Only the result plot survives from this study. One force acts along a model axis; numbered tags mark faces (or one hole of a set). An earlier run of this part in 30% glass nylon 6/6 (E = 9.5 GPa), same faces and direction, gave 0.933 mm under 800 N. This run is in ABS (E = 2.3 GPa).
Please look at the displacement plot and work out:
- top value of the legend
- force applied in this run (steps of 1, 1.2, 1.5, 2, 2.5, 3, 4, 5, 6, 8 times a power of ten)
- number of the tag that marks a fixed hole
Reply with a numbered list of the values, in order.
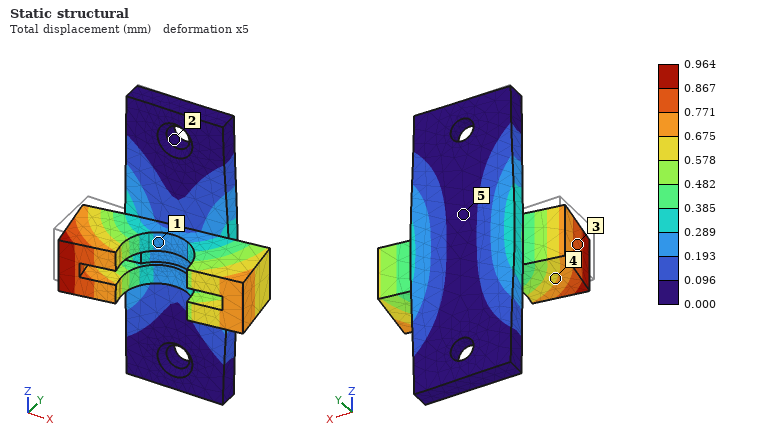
1. 0.964 mm
2. 200 N
3. 2
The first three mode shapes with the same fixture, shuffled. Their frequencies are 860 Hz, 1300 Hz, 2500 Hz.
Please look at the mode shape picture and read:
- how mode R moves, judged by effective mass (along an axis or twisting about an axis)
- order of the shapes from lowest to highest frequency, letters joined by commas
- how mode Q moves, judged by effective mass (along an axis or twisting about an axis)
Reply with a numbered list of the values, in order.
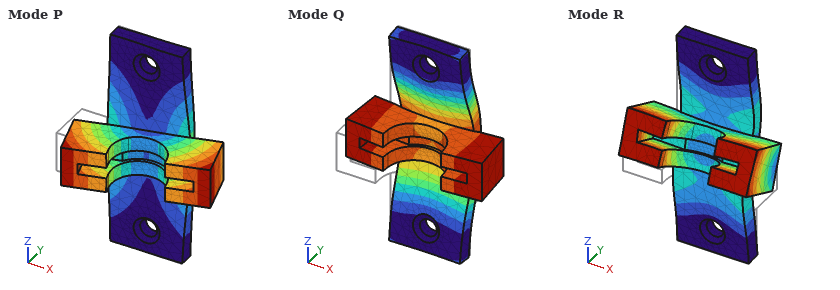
1. along Z
2. P, Q, R
3. along Y
